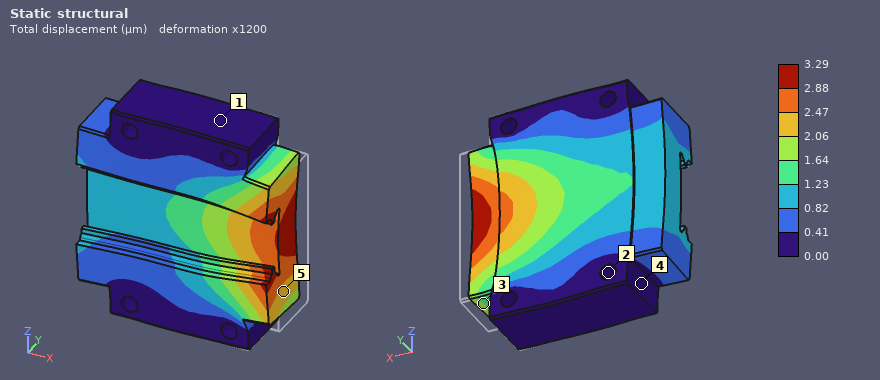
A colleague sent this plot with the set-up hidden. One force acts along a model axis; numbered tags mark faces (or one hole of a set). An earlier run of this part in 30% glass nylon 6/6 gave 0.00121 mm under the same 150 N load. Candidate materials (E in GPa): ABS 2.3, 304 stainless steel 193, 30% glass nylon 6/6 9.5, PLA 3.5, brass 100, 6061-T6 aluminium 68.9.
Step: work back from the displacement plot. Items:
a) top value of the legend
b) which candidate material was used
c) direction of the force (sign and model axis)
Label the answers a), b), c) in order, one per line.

a) 3.29 µm
b) PLA
c) -X
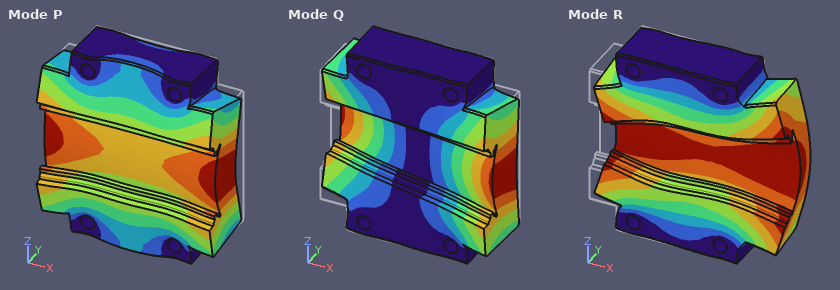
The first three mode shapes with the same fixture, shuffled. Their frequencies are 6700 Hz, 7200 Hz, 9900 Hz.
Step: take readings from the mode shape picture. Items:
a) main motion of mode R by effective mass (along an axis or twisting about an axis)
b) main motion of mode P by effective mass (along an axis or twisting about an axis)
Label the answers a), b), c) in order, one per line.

a) along X
b) along Y
